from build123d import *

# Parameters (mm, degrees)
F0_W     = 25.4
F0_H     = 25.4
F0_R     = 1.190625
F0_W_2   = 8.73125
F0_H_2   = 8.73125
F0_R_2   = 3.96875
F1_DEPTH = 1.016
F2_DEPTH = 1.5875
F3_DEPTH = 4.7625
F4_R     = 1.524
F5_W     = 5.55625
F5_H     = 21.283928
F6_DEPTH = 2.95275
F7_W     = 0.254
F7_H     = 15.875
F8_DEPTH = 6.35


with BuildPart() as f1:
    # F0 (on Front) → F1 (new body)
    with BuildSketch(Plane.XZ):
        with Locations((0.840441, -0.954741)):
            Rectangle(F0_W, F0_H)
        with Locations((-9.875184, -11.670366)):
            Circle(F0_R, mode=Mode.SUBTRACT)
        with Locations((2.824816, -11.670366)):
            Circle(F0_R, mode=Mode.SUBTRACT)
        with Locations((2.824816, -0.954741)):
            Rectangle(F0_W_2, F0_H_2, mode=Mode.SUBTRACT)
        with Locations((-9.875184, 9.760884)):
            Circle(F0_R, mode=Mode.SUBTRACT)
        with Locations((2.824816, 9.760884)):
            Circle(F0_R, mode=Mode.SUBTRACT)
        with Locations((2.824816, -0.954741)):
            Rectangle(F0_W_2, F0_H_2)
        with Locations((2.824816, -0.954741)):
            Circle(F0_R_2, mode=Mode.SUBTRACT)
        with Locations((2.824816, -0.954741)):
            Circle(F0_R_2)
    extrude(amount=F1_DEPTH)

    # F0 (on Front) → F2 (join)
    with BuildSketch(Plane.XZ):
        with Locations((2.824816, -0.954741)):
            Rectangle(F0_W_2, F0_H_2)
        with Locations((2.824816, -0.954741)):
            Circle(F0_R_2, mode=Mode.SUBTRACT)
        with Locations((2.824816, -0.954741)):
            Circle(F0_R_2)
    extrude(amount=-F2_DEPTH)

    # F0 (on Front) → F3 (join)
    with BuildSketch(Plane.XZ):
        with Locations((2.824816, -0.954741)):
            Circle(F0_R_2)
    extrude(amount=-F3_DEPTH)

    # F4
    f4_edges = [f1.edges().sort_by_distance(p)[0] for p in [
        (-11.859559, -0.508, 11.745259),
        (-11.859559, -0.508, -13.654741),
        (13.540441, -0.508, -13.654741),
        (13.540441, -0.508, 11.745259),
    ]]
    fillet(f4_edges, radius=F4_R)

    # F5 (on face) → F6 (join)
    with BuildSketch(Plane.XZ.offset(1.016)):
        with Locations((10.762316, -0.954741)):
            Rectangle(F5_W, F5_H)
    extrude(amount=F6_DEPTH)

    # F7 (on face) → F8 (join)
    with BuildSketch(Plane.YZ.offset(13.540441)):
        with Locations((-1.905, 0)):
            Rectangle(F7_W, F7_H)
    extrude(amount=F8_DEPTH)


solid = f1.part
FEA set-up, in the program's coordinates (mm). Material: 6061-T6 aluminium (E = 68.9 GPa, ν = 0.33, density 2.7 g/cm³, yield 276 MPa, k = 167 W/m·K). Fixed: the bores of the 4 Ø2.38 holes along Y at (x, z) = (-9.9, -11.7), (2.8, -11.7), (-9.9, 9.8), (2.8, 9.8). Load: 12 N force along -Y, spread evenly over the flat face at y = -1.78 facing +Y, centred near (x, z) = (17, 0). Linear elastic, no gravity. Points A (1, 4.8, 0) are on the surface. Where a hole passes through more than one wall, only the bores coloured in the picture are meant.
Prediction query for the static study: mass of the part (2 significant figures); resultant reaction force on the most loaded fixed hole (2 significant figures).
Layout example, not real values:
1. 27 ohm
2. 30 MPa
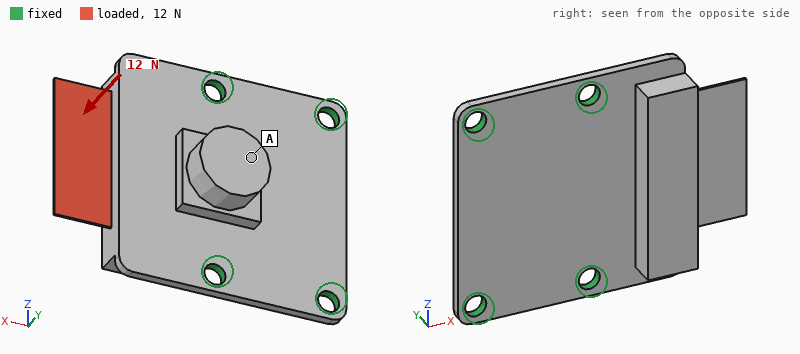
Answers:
1. 3.5 g
2. 10 N
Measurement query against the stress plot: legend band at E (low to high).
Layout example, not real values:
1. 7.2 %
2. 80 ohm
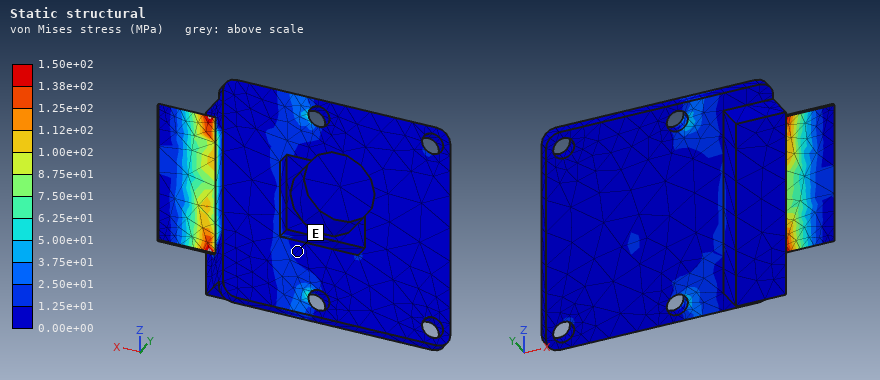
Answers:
1. 0.00e+00 to 1.25e+01 MPa
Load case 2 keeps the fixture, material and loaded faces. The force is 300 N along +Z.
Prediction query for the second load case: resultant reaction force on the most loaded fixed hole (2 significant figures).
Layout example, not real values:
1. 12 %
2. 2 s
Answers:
1. 230 N
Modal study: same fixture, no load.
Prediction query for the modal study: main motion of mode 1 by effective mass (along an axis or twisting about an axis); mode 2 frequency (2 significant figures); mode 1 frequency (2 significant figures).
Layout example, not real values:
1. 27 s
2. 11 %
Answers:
1. along Y
2. 6000 Hz
3. 4000 Hz
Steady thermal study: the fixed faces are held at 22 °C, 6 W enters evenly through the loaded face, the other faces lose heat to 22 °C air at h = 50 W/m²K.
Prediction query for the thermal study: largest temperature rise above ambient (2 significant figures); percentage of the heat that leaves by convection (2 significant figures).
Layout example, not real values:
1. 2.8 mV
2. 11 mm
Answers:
1. 41 K
2. 9.9 %
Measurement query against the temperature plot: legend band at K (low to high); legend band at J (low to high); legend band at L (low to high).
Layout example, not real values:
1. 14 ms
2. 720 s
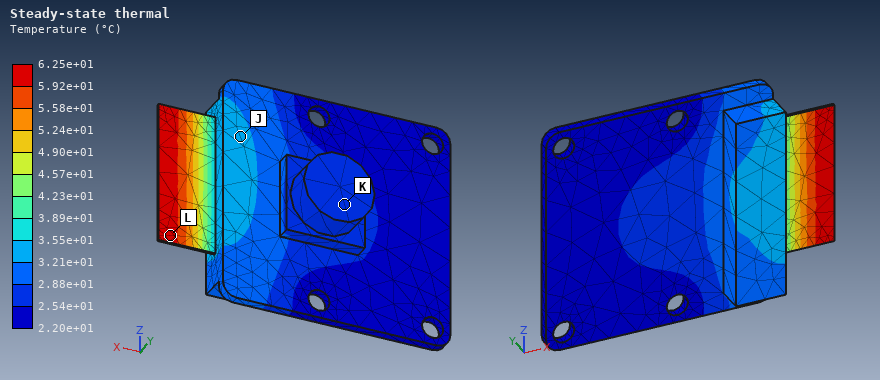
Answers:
1. 2.54e+01 to 2.88e+01 °C
2. 3.21e+01 to 3.55e+01 °C
3. 5.92e+01 to 6.25e+01 °C
